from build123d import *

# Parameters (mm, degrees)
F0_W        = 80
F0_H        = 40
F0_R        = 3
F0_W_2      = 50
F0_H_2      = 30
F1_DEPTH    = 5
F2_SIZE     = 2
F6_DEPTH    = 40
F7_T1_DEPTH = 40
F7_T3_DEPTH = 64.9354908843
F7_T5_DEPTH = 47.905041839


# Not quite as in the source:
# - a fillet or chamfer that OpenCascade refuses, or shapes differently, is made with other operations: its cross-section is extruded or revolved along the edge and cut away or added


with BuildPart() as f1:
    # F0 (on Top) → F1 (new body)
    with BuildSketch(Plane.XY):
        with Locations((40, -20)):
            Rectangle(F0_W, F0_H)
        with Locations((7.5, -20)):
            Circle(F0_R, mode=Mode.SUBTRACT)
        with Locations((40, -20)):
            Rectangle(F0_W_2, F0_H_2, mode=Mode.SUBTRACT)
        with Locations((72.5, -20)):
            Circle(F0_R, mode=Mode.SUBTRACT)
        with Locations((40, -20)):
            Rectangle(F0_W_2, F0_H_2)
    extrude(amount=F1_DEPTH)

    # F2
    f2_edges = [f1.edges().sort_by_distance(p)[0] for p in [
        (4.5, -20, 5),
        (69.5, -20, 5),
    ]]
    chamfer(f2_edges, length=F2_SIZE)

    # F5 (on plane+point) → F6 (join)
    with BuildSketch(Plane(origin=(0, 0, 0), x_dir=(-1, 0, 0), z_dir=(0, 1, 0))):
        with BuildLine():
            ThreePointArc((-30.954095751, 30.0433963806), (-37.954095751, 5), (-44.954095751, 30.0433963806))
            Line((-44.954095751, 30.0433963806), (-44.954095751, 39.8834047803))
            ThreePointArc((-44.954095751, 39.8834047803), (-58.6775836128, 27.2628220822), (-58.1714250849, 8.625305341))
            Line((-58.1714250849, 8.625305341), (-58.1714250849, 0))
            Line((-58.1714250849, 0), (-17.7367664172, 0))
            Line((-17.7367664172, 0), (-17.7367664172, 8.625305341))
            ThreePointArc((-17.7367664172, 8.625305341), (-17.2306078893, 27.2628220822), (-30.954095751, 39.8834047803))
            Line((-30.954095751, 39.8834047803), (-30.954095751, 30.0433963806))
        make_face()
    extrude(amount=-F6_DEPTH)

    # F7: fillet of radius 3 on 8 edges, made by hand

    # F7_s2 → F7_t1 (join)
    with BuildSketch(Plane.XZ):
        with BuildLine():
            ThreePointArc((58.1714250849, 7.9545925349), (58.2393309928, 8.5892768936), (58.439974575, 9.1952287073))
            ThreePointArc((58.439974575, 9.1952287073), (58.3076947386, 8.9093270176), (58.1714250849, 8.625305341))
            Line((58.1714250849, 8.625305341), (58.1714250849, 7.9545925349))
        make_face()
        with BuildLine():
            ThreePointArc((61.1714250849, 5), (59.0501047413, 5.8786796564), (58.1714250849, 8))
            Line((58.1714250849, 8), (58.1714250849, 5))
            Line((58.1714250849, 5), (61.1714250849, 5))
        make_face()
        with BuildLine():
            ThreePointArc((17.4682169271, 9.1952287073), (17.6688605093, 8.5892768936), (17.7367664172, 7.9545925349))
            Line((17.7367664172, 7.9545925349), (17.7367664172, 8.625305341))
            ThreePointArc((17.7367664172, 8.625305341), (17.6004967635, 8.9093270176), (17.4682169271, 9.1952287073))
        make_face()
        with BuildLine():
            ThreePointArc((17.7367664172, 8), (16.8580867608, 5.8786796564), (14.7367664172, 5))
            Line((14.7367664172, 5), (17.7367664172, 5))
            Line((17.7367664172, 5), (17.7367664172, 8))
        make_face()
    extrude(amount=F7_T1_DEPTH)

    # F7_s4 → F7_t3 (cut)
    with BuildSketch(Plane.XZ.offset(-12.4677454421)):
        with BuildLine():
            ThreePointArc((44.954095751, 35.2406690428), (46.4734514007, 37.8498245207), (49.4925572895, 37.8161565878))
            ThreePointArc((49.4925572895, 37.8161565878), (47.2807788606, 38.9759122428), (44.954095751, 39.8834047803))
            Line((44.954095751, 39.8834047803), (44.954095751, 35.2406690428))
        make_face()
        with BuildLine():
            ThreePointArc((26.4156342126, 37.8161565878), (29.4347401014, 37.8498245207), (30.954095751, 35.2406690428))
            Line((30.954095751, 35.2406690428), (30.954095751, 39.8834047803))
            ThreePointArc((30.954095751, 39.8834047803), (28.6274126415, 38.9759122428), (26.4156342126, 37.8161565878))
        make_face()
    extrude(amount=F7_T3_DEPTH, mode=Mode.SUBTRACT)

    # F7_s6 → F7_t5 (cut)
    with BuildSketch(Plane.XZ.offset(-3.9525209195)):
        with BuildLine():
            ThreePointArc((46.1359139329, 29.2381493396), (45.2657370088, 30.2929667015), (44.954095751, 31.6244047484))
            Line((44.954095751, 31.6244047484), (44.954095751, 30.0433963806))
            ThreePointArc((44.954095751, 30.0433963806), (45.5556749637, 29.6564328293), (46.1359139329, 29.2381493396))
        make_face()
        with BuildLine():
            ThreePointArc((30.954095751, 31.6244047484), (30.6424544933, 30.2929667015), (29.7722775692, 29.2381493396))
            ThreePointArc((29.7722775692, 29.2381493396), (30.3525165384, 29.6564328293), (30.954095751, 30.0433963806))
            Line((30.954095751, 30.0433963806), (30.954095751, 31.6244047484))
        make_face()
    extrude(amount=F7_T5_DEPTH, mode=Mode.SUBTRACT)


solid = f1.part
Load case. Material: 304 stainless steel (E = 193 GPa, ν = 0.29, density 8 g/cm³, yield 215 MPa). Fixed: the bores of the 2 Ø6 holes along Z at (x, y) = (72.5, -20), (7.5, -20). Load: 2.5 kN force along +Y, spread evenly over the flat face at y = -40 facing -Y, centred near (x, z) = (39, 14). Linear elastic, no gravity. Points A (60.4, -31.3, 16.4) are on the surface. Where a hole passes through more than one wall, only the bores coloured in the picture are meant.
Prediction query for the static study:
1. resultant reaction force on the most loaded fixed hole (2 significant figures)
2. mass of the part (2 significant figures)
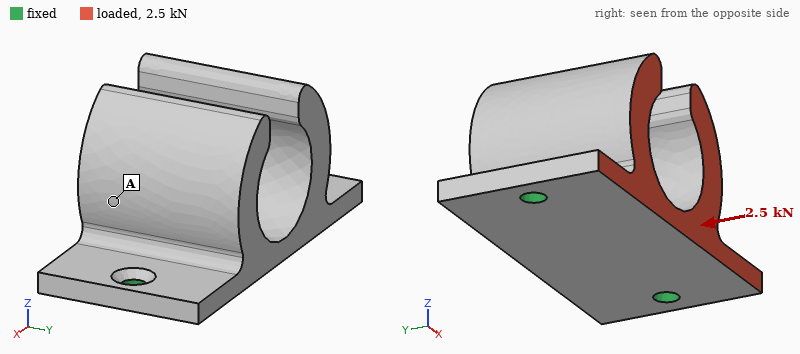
1.3 kN
340 g
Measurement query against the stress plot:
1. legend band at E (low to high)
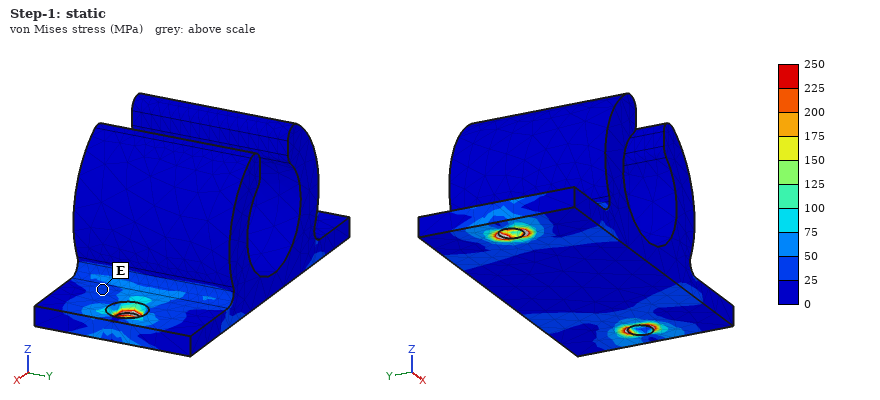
25 to 50 MPa
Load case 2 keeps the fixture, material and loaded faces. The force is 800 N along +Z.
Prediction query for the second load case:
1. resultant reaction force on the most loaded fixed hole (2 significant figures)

550 N
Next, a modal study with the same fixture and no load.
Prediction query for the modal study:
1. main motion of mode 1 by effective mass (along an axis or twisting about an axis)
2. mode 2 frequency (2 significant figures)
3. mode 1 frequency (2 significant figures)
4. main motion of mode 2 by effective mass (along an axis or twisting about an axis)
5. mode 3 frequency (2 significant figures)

along Y
2300 Hz
1600 Hz
along Z
4200 Hz
